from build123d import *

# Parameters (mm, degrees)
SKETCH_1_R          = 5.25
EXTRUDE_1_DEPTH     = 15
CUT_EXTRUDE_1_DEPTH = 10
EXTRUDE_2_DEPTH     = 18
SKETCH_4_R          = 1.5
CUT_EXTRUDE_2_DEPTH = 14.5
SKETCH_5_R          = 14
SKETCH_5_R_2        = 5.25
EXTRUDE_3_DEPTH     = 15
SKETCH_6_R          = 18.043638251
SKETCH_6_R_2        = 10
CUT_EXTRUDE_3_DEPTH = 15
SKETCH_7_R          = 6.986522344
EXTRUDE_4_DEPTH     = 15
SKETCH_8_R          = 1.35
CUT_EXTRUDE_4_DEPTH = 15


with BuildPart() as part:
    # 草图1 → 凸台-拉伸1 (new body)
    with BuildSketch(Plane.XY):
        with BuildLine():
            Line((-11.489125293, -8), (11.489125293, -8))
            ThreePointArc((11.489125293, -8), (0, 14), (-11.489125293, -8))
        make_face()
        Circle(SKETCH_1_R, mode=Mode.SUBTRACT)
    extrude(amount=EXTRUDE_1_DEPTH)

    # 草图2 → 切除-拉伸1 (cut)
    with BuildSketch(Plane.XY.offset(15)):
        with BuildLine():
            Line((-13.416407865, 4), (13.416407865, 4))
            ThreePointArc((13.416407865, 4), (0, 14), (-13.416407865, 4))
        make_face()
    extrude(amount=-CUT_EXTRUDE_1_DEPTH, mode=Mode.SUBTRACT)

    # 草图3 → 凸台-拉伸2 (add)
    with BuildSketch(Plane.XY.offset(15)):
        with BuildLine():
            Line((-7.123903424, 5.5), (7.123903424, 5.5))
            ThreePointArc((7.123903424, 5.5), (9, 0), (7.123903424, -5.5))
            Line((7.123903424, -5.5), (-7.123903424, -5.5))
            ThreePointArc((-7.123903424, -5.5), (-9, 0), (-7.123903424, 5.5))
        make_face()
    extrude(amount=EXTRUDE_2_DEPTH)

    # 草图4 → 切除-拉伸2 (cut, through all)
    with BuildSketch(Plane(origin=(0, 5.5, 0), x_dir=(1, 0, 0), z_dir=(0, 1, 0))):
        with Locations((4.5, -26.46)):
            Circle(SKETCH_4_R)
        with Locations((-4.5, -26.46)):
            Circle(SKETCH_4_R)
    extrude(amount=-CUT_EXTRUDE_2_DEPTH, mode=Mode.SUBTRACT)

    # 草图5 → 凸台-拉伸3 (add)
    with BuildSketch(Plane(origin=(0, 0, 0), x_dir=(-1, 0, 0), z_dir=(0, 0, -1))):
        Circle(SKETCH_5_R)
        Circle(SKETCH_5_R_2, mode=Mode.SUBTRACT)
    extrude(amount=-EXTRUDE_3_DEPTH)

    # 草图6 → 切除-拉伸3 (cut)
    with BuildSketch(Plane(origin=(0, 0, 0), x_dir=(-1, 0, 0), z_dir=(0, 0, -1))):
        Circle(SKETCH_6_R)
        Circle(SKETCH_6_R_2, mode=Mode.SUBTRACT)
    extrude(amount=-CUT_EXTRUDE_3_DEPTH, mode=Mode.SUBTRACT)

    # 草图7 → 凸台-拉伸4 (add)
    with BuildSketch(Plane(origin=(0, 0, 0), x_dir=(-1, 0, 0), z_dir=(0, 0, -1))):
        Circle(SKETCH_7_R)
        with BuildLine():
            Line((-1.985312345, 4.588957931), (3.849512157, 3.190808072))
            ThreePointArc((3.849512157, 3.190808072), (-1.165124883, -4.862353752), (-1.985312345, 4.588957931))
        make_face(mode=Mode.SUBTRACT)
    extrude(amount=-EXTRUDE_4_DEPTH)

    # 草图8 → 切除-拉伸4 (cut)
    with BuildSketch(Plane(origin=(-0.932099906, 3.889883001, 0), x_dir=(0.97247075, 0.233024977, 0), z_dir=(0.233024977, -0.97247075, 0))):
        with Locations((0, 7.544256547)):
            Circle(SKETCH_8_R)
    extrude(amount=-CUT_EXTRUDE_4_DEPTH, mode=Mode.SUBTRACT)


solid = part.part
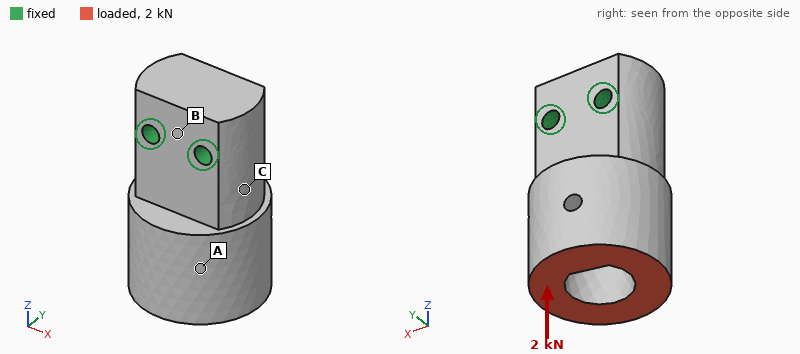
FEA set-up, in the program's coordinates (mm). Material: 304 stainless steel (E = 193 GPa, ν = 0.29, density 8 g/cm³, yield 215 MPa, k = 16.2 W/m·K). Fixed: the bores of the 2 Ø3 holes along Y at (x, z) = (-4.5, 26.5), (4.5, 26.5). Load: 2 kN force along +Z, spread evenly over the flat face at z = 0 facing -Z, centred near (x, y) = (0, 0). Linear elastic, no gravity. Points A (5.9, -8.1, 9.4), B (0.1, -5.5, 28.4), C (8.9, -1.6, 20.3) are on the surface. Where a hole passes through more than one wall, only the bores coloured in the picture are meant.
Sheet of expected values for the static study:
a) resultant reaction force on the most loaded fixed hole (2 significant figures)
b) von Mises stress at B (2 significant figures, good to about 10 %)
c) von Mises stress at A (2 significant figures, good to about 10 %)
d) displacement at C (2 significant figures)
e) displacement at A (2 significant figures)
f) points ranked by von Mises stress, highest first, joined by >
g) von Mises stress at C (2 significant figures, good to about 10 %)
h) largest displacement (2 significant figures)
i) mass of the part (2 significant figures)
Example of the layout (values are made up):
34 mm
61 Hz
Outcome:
1.0 kN
3.3 MPa
7.4 MPa
0.42 µm
1.1 µm
C > A > B
11 MPa
1.7 µm
54 g
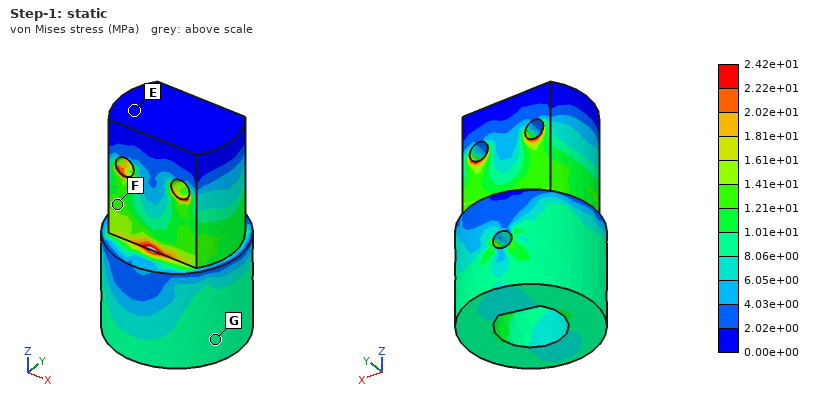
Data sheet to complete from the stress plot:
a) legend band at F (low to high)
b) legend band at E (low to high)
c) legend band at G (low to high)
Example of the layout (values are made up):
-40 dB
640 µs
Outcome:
1.21e+01 to 1.41e+01 MPa
0.00e+00 to 2.02e+00 MPa
8.06e+00 to 1.01e+01 MPa
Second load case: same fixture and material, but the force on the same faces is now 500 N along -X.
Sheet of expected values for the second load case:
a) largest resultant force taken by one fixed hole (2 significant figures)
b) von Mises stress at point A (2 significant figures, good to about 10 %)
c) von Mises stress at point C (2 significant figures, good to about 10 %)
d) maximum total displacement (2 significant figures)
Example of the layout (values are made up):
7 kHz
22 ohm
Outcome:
1.2 kN
4.7 MPa
20 MPa
5.8 µm
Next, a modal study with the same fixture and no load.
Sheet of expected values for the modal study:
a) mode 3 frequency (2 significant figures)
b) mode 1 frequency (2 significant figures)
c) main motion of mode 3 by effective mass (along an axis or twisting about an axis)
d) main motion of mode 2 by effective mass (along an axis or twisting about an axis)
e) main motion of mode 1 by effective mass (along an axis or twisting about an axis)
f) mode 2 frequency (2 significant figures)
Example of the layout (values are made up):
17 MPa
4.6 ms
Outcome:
20 kHz
9200 Hz
twisting about Z
along X
along Y
13 kHz
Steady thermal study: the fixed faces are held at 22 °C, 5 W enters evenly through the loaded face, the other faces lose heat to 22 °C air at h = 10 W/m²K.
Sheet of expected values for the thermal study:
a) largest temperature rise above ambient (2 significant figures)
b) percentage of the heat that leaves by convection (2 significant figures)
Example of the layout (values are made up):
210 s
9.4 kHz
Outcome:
39 K
10 %
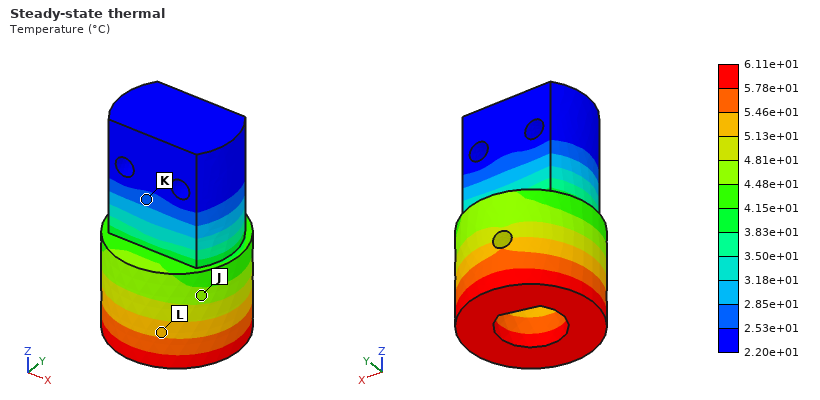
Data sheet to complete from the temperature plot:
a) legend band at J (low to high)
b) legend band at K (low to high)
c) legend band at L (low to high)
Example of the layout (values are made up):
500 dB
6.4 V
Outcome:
4.48e+01 to 4.81e+01 °C
2.53e+01 to 2.85e+01 °C
5.13e+01 to 5.46e+01 °C
